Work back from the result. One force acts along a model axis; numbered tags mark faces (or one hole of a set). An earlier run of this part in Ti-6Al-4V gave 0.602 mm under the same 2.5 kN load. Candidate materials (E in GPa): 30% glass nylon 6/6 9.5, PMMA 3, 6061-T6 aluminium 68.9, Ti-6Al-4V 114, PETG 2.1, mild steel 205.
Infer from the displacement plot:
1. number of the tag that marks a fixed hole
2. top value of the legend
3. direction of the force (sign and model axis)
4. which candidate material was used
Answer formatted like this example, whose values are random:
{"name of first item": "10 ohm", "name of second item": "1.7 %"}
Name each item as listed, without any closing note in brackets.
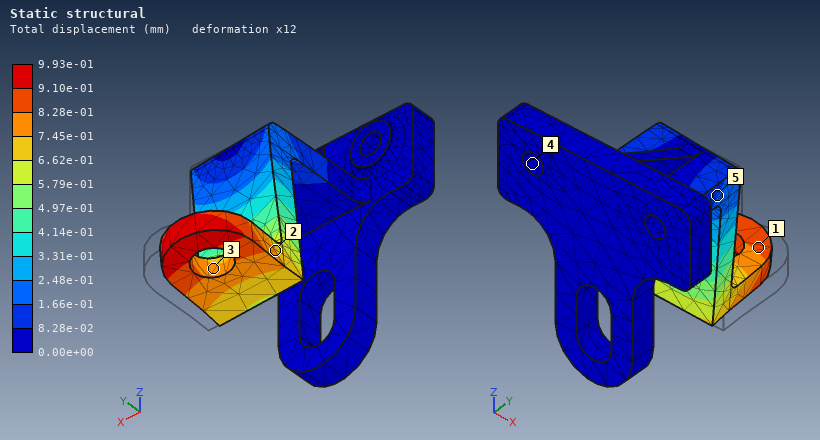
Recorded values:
{"number of the tag that marks a fixed hole": "4", "top value of the legend": "9.93e-01 mm", "direction of the force": "-X", "which candidate material was used": "6061-T6 aluminium"}
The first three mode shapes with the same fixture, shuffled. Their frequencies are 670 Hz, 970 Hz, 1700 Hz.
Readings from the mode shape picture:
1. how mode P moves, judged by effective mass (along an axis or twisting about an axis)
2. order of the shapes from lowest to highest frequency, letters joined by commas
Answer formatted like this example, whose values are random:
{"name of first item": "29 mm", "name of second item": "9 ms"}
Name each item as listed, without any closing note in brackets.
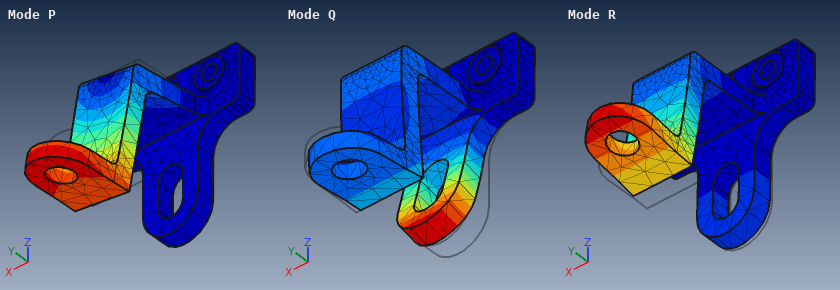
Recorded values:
{"how mode P moves, judged by effective mass": "along X", "order of the shapes from lowest to highest frequency, letters joined by commas": "R, P, Q"}
